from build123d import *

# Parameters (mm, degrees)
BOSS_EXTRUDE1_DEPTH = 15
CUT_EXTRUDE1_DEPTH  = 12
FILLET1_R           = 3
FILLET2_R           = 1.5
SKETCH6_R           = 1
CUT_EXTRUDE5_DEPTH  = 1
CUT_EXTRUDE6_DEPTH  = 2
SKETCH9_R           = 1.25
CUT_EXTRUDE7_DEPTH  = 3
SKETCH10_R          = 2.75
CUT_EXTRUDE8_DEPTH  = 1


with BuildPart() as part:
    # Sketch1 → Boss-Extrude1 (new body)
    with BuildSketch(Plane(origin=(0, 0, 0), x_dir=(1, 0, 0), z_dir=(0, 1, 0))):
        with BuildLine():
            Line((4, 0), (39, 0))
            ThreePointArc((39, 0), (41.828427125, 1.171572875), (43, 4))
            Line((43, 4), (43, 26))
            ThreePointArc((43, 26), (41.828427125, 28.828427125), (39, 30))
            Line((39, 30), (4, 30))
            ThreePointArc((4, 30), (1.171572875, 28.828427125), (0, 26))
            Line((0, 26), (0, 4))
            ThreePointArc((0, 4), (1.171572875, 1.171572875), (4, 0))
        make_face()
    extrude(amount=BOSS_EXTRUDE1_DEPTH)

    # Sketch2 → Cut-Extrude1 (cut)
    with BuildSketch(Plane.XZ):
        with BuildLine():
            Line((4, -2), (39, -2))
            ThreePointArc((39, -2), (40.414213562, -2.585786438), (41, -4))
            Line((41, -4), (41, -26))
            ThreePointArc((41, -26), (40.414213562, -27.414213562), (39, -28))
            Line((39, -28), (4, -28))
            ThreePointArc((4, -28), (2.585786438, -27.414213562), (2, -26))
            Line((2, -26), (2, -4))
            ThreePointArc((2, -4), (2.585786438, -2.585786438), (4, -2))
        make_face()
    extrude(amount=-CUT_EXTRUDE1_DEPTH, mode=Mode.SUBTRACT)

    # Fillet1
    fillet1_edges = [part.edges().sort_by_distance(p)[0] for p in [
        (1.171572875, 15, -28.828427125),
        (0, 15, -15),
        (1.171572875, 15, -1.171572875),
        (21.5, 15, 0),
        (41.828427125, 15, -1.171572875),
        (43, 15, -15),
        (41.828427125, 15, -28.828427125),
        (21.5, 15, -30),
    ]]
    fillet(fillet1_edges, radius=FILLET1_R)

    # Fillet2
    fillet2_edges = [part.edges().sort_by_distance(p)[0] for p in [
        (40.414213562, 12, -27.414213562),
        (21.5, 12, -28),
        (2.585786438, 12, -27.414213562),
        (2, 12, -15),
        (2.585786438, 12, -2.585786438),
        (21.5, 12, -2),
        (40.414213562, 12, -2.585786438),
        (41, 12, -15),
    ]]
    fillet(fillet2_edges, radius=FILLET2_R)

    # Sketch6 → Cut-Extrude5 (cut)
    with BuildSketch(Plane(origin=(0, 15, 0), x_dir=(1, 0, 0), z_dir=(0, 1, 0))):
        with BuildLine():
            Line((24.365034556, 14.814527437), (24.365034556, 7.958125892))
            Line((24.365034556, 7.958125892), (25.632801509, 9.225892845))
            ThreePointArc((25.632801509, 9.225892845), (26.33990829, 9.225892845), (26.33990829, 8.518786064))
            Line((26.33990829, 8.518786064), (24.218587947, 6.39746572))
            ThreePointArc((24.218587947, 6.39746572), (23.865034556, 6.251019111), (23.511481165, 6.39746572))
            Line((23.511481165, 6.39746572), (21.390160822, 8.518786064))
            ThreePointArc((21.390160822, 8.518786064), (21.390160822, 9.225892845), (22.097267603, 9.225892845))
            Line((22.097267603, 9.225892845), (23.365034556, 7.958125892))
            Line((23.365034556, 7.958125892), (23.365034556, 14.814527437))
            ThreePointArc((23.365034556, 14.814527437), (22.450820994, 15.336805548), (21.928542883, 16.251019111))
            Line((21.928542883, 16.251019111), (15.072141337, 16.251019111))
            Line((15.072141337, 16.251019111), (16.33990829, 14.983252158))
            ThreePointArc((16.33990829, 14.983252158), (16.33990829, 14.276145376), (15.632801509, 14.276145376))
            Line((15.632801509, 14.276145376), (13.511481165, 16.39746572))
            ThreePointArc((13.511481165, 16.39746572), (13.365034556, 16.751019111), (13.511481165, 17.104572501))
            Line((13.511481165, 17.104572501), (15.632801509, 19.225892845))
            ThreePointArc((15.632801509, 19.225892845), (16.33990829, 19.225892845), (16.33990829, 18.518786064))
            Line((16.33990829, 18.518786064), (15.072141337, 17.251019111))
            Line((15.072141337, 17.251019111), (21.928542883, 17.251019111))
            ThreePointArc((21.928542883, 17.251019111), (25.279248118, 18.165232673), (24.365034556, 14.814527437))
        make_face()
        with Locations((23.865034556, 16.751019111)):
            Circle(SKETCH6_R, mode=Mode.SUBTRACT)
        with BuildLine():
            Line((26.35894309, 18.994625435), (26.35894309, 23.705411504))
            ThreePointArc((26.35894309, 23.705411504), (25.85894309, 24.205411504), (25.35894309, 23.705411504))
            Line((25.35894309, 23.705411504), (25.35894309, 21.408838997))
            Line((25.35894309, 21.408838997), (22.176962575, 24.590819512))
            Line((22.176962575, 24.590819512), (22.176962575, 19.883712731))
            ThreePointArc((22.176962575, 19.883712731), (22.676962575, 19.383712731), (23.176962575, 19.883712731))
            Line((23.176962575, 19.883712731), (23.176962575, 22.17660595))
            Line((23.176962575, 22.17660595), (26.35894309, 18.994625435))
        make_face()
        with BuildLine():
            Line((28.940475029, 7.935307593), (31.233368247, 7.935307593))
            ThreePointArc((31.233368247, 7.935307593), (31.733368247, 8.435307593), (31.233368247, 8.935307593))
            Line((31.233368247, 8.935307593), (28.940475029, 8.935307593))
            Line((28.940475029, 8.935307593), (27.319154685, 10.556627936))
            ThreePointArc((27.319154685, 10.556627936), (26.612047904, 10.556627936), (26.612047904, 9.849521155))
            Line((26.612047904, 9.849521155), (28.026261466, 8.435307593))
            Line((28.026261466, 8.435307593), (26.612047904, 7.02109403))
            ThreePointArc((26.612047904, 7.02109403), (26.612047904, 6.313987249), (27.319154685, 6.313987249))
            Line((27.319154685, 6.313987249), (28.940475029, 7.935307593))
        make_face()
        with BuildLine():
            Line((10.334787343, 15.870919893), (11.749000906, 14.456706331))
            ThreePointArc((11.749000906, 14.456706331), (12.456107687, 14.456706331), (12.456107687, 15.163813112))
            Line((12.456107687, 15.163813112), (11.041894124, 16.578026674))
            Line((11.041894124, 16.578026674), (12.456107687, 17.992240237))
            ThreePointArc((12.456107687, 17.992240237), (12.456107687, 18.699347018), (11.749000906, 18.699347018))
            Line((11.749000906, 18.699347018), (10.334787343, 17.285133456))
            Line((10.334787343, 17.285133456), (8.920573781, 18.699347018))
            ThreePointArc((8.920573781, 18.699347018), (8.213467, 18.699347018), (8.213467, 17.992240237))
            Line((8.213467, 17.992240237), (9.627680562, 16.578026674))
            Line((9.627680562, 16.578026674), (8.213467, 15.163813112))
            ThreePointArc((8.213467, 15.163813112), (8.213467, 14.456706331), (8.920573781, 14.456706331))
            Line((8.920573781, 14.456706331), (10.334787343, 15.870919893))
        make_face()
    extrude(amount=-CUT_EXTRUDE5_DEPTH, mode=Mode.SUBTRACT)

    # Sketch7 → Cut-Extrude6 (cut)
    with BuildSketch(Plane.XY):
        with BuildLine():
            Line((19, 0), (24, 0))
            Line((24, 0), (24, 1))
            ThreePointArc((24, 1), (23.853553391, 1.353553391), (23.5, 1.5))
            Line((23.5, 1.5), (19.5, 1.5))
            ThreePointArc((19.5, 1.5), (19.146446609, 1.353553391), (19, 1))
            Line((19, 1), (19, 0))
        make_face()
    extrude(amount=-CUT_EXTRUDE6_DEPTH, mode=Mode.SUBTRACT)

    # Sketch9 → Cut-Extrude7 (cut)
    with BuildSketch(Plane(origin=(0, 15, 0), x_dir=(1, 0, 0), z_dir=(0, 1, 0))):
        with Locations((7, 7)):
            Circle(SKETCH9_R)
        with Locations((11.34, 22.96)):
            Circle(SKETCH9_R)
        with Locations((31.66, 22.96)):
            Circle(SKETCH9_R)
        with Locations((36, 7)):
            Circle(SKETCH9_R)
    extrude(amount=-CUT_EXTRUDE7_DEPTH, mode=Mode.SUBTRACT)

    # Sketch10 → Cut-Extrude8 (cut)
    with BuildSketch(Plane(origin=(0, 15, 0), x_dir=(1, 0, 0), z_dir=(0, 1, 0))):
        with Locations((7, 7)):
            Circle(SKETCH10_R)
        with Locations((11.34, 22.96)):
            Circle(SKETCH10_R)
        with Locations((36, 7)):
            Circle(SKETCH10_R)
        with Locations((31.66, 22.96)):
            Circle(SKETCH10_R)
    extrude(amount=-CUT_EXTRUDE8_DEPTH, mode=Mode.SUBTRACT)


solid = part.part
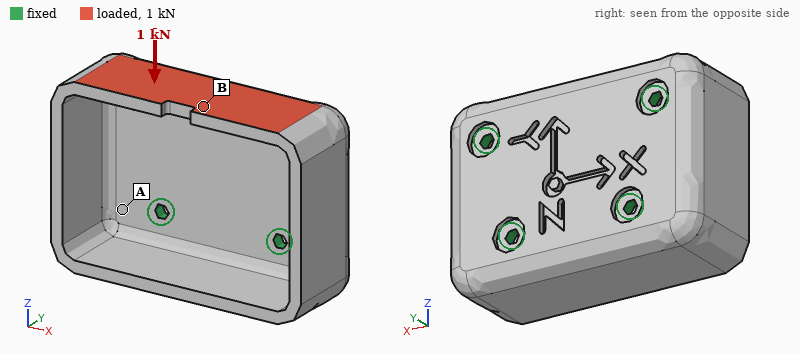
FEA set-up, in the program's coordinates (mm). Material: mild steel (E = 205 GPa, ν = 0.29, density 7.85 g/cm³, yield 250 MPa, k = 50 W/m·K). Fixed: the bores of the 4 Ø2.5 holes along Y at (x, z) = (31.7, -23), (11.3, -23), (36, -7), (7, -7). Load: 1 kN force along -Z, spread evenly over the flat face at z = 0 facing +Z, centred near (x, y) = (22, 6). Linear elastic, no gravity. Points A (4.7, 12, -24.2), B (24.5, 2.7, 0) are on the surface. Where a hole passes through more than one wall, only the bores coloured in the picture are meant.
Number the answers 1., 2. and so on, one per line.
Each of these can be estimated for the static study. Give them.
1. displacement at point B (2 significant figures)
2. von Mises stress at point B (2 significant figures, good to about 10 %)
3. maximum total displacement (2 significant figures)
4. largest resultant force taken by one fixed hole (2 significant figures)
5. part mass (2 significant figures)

1. 39 µm
2. 45 MPa
3. 50 µm
4. 390 N
5. 52 g
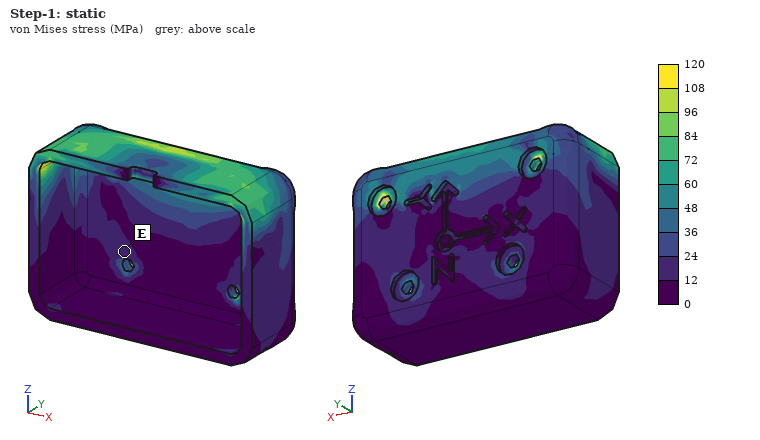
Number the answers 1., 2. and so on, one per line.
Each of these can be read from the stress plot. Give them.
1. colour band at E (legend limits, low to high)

1. 12 to 24 MPa
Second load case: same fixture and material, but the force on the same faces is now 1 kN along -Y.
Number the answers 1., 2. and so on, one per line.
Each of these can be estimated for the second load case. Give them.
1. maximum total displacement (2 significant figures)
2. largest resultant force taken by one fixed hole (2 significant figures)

1. 23 µm
2. 650 N
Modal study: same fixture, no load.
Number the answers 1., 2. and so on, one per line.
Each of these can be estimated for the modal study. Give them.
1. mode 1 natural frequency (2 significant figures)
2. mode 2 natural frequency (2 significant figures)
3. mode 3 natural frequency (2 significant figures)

1. 10 kHz
2. 10 kHz
3. 11 kHz
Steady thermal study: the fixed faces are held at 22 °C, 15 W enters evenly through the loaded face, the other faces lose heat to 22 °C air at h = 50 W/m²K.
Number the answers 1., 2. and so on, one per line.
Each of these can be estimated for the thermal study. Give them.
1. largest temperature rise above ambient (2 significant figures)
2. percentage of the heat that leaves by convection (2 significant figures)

1. 41 K
2. 17 %
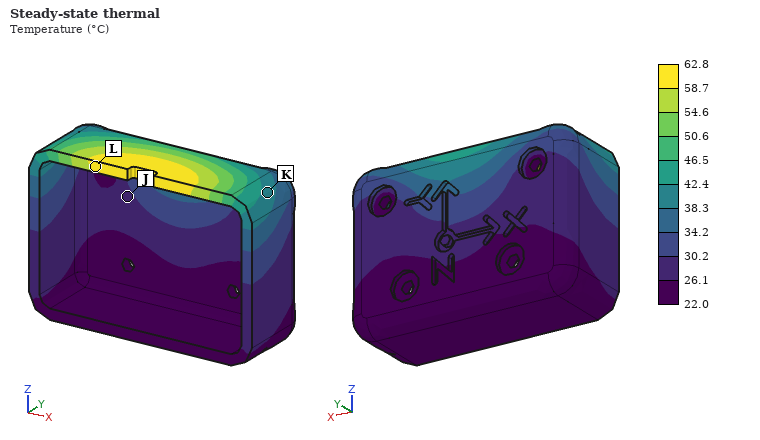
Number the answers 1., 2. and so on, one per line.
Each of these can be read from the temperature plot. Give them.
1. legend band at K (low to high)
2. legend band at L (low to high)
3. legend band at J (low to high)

1. 38.3 to 42.4 °C
2. 58.7 to 62.8 °C
3. 26.1 to 30.2 °C
